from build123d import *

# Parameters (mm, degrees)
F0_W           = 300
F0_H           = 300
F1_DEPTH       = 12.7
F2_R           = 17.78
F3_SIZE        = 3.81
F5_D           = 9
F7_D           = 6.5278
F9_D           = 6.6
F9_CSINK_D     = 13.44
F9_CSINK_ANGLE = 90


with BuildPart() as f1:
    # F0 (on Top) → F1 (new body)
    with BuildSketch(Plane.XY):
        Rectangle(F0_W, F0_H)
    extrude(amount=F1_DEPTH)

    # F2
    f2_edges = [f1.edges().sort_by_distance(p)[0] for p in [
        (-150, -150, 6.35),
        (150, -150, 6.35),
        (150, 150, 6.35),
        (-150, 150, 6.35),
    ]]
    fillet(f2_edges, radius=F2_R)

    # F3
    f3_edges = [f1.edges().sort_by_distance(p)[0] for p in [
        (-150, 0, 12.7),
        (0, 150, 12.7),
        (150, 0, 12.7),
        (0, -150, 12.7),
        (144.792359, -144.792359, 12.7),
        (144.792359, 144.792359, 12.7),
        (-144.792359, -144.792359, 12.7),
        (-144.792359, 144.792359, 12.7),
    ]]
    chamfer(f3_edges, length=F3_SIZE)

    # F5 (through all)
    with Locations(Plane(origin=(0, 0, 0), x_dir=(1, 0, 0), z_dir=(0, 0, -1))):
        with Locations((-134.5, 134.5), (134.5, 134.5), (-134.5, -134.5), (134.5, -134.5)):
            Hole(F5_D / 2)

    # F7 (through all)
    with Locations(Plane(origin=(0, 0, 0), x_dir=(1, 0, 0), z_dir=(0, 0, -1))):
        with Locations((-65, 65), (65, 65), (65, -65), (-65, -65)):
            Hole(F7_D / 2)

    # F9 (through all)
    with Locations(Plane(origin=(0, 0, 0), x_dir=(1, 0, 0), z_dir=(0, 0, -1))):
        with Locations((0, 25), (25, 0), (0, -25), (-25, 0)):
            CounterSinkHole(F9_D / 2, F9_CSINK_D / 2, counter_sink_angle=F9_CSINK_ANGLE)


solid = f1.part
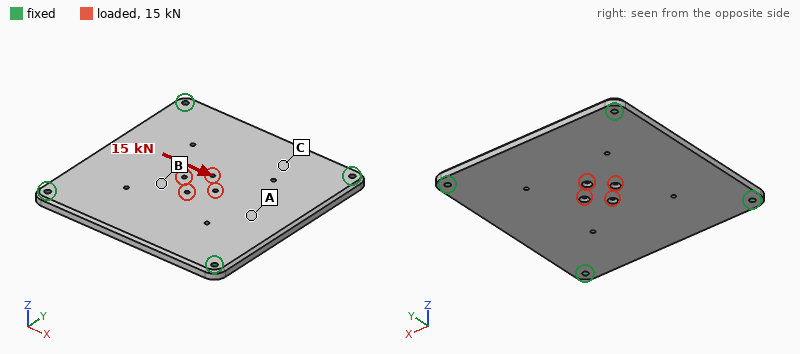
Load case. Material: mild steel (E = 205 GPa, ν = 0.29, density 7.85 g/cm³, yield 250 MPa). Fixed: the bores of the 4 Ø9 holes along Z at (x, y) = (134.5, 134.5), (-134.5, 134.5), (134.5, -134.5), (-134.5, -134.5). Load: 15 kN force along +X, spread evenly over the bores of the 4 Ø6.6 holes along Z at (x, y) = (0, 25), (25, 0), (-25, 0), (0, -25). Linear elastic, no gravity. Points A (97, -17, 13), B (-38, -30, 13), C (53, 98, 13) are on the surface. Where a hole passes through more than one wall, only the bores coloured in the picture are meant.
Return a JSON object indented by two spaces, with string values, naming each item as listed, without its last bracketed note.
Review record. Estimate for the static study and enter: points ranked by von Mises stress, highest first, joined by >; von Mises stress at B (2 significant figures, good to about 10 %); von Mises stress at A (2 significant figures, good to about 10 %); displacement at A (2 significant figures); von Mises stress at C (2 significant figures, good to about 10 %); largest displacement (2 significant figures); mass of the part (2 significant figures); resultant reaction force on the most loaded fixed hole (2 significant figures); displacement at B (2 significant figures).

{
  "points ranked by von Mises stress, highest first, joined by >": "B > C > A",
  "von Mises stress at B": "6.2 MPa",
  "von Mises stress at A": "1.9 MPa",
  "displacement at A": "5.4 µm",
  "von Mises stress at C": "4.3 MPa",
  "largest displacement": "7.4 µm",
  "mass of the part": "8.8 kg",
  "resultant reaction force on the most loaded fixed hole": "4.3 kN",
  "displacement at B": "5.6 µm"
}
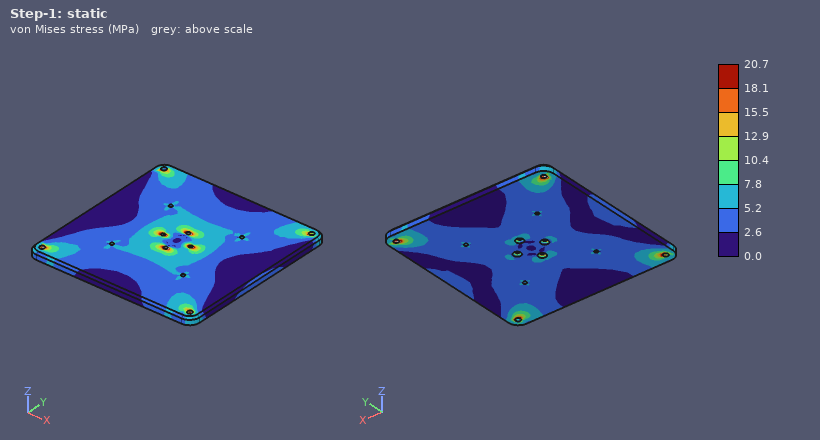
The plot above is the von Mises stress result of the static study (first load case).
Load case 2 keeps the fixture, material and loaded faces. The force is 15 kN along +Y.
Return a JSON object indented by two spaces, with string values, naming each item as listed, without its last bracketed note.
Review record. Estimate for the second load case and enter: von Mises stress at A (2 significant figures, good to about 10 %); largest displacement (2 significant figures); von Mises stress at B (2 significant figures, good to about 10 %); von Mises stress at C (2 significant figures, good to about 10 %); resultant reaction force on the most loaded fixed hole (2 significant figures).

{
  "von Mises stress at A": "3.7 MPa",
  "largest displacement": "7.4 µm",
  "von Mises stress at B": "6.5 MPa",
  "von Mises stress at C": "3.4 MPa",
  "resultant reaction force on the most loaded fixed hole": "4.3 kN"
}
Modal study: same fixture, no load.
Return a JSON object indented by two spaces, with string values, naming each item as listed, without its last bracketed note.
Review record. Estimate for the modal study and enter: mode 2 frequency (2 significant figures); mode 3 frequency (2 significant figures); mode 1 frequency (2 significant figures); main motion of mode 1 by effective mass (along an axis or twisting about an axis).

{
  "mode 2 frequency": "950 Hz",
  "mode 3 frequency": "950 Hz",
  "mode 1 frequency": "530 Hz",
  "main motion of mode 1 by effective mass": "along Z"
}
